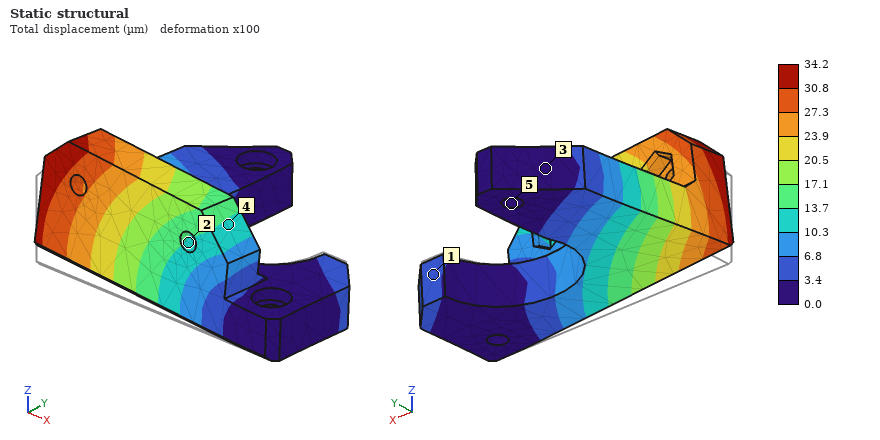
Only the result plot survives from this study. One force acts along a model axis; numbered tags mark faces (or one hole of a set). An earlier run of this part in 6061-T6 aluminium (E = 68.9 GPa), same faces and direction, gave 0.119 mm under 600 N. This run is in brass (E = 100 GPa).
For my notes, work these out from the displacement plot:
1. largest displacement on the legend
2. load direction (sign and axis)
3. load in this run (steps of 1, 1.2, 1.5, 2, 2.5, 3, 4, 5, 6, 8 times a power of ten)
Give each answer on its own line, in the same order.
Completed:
34.2 µm
+Z
250 N
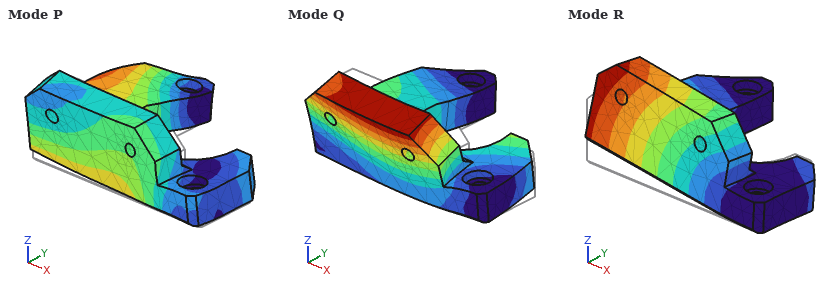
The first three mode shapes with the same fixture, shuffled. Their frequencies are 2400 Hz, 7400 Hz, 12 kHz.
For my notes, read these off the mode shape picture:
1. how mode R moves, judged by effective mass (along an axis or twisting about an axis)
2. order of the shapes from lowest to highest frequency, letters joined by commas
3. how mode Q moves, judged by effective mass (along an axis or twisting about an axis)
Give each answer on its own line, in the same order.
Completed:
along Z
R, Q, P
along Y
